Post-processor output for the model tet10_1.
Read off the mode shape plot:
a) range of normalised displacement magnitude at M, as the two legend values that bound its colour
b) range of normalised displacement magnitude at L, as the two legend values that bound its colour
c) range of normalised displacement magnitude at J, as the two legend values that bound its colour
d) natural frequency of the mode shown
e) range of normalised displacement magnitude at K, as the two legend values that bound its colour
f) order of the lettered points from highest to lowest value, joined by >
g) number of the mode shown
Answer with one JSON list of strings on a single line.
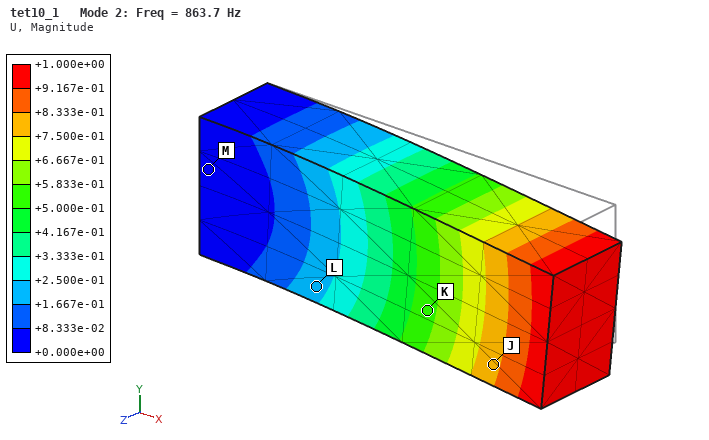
["+0.000e+00 to +8.333e-02", "+1.667e-01 to +2.500e-01", "+7.500e-01 to +8.333e-01", "863.7 Hz", "+5.000e-01 to +5.833e-01", "J > K > L > M", "2"]
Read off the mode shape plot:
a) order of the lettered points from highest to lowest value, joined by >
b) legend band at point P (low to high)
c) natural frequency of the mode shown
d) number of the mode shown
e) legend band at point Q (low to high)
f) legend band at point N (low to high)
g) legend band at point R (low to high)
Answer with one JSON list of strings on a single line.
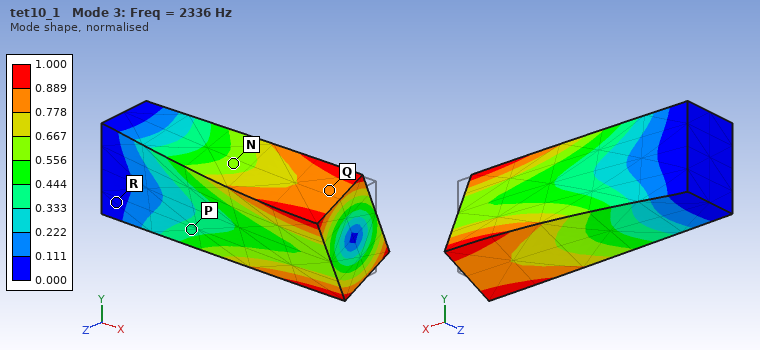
["Q > N > P > R", "0.333 to 0.444", "2336 Hz", "3", "0.778 to 0.889", "0.556 to 0.667", "0.000 to 0.111"]
